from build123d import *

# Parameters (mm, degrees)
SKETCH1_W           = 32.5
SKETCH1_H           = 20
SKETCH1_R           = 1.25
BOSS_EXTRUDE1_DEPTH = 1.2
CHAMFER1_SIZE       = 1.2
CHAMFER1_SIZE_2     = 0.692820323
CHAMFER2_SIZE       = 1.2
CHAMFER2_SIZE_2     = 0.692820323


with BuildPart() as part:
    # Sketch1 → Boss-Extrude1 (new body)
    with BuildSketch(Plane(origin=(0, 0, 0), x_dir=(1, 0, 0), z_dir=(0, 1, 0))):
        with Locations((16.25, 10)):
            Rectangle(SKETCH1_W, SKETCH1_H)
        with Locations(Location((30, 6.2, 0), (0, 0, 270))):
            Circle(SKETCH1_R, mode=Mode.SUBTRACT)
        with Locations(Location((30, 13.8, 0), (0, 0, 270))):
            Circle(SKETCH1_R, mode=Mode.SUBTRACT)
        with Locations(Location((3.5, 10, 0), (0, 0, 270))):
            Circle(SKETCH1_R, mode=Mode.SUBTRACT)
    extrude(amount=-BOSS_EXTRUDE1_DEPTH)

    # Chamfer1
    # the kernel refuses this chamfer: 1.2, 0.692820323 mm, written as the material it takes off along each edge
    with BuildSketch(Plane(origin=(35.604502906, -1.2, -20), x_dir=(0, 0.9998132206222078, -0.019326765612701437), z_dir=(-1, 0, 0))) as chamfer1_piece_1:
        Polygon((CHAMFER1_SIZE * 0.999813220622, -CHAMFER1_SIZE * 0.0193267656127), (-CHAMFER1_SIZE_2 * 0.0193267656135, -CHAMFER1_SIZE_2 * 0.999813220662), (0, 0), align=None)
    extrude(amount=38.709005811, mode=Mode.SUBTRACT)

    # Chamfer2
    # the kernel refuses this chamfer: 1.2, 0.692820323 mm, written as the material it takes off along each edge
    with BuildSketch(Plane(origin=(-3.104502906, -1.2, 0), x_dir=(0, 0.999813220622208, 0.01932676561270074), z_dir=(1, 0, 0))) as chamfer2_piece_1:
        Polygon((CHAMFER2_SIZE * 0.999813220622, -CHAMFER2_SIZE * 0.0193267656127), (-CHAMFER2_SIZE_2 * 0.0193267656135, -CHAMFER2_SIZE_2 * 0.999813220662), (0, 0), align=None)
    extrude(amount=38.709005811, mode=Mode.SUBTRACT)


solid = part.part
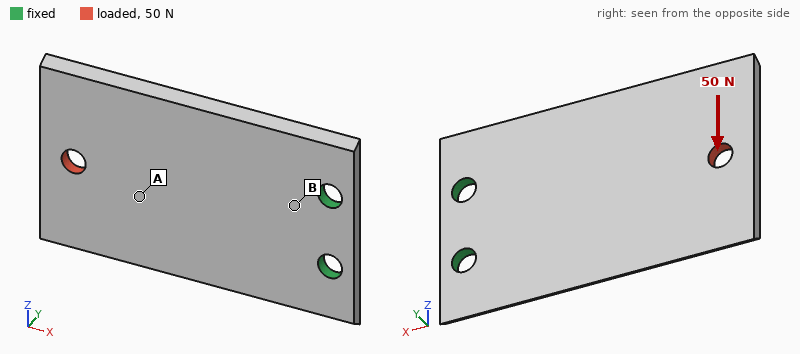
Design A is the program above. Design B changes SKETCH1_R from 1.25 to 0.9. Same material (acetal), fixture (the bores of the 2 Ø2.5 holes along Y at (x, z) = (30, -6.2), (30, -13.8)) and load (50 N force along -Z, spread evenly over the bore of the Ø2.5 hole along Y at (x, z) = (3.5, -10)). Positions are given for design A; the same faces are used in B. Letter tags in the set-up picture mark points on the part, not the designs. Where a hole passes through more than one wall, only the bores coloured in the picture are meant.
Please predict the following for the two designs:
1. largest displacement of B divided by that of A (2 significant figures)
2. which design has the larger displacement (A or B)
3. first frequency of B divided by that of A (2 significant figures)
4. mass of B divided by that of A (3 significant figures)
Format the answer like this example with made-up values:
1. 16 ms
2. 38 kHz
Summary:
1. 1.2
2. B
3. 0.96
4. 1.01
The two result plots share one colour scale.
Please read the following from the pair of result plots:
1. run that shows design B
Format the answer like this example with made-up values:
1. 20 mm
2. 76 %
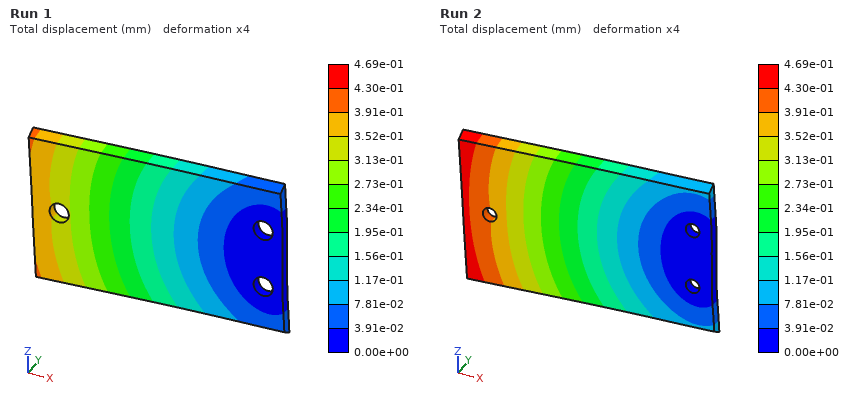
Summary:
1. Run 2
